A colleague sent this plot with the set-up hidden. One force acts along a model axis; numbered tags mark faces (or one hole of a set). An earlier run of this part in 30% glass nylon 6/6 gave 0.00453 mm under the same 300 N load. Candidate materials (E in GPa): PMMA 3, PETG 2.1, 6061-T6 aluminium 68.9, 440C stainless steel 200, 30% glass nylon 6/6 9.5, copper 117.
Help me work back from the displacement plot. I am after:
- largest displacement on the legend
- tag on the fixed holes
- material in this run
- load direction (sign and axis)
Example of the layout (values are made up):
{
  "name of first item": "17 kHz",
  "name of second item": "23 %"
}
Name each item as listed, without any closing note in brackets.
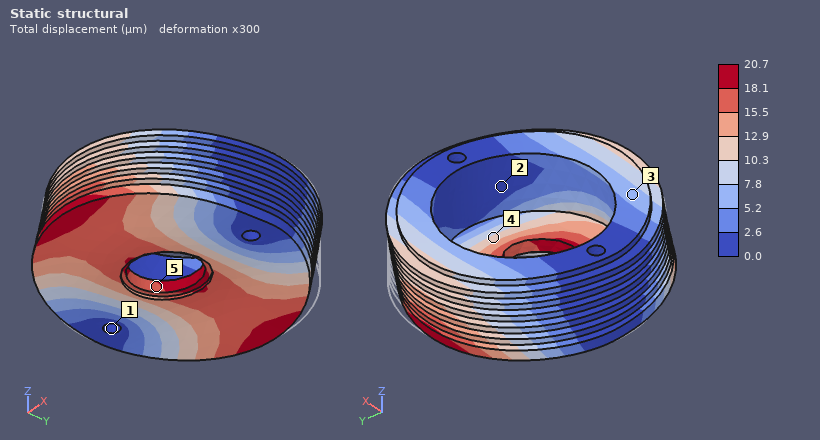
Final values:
{
  "largest displacement on the legend": "20.7 µm",
  "tag on the fixed holes": "1",
  "material in this run": "PETG",
  "load direction": "-Y"
}
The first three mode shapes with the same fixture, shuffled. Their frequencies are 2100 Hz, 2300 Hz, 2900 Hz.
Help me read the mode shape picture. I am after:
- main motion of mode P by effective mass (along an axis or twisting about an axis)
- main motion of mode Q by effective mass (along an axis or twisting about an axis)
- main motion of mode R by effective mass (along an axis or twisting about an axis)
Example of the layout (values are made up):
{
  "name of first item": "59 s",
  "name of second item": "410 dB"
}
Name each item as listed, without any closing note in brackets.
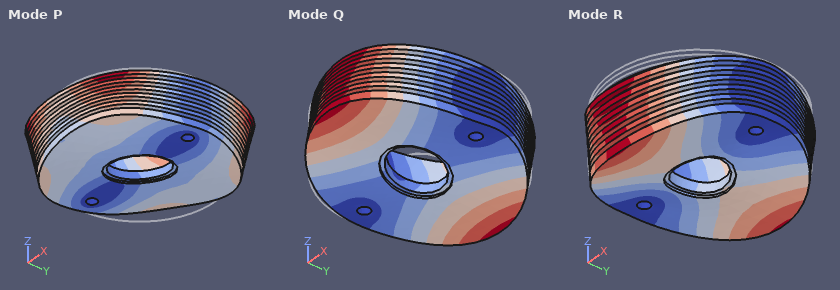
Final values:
{
  "main motion of mode P by effective mass": "twisting about Z",
  "main motion of mode Q by effective mass": "twisting about X",
  "main motion of mode R by effective mass": "along Z"
}
